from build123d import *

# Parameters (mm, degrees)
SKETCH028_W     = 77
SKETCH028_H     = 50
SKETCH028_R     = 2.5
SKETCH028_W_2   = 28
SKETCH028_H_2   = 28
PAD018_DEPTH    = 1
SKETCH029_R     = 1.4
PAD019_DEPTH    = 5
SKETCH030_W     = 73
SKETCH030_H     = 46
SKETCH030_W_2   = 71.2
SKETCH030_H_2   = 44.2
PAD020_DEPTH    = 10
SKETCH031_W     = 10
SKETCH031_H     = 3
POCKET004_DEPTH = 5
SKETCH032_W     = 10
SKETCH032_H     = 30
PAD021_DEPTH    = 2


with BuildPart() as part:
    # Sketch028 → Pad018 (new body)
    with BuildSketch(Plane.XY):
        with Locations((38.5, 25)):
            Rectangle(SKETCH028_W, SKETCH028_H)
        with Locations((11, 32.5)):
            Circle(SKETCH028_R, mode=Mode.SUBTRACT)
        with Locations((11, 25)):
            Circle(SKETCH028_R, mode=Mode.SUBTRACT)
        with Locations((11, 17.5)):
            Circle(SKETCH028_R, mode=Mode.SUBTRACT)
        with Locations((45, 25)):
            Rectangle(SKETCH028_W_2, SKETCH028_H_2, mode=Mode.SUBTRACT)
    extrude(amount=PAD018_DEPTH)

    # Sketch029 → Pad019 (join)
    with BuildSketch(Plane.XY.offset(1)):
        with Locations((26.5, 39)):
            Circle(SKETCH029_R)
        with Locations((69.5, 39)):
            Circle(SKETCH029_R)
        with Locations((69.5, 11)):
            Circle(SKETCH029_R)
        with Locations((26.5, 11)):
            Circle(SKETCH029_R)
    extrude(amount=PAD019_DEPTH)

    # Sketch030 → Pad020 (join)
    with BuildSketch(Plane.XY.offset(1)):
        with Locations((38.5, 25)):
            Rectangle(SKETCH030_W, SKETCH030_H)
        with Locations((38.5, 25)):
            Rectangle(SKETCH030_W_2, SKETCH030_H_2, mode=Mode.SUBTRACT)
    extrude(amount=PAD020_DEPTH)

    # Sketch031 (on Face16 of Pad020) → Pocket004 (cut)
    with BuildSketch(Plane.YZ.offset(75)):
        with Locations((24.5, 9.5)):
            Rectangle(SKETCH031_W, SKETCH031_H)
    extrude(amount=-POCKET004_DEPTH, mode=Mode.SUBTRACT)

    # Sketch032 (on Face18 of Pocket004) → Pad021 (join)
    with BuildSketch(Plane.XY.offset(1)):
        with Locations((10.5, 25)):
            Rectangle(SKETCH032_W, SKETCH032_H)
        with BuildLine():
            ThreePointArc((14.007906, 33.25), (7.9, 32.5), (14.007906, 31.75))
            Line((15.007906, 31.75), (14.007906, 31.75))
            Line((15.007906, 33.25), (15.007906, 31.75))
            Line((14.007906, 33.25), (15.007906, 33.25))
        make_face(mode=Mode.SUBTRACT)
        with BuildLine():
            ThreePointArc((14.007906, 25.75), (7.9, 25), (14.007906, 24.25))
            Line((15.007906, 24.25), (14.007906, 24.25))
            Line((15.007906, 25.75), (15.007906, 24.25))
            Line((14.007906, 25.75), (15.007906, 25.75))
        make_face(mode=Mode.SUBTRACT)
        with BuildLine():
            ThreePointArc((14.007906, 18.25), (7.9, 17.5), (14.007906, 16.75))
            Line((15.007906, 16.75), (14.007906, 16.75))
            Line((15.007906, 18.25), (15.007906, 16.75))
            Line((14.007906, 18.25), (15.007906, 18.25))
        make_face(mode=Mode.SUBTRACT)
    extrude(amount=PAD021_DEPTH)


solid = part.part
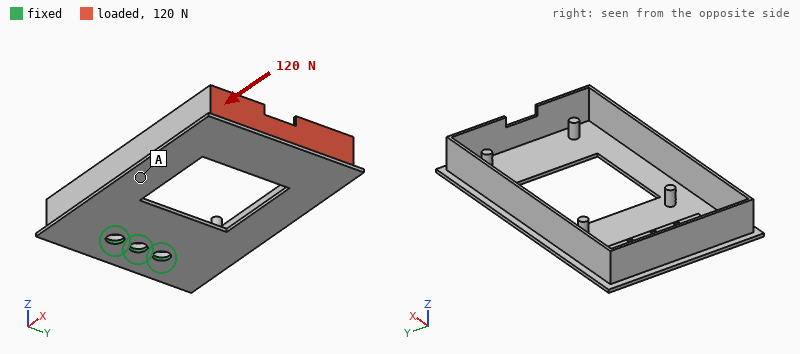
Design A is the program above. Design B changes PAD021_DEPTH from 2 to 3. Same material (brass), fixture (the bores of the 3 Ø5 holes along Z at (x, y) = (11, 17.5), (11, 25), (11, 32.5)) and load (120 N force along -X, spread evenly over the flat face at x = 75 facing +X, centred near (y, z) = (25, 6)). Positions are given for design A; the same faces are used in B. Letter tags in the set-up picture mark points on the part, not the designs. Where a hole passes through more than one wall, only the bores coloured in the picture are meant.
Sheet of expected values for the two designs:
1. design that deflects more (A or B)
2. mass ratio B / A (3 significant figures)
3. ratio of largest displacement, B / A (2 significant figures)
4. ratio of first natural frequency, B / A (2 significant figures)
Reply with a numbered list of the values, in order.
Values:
1. A
2. 1.04
3. 0.92
4. 1.1
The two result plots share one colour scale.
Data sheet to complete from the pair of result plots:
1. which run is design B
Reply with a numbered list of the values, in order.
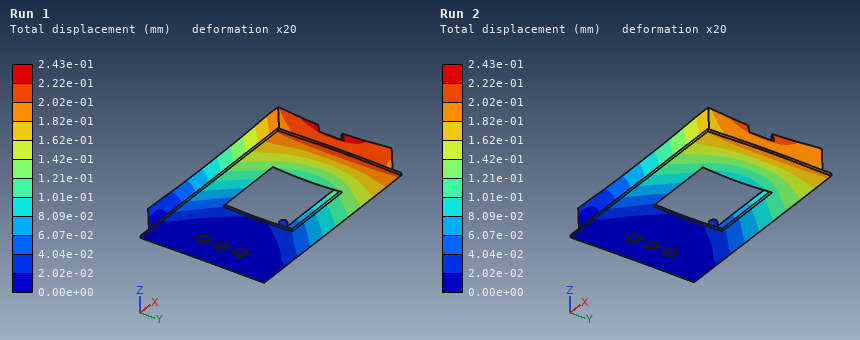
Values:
1. Run 2
